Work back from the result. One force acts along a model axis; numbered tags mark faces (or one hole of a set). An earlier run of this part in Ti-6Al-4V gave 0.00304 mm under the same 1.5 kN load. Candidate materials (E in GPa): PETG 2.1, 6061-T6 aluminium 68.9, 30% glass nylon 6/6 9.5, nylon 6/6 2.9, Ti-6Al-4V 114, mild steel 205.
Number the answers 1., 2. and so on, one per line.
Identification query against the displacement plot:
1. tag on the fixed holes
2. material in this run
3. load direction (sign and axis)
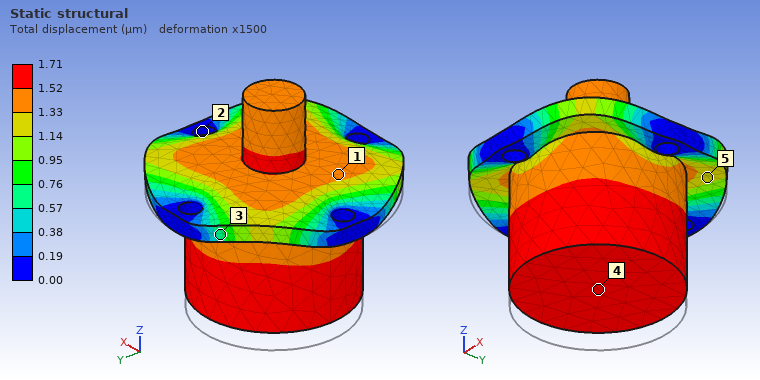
1. 2
2. mild steel
3. +Z
